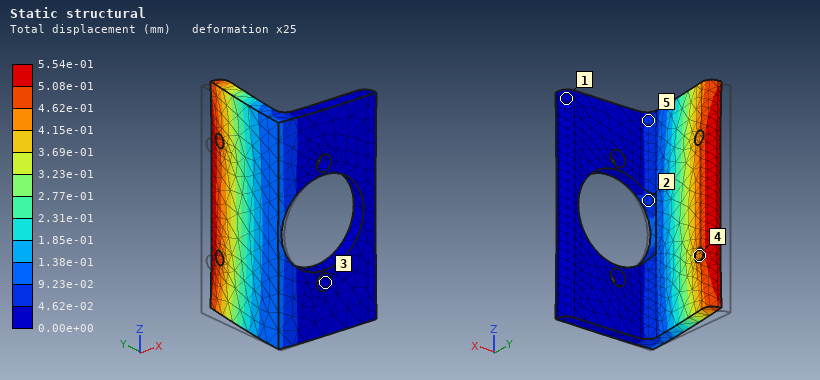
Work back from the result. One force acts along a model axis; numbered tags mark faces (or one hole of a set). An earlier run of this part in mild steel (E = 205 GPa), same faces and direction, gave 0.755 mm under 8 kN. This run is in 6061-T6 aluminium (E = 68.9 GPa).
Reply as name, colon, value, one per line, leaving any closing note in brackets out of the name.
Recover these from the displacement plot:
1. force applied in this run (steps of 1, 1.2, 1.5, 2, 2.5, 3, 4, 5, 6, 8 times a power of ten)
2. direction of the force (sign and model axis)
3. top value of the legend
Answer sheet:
force applied in this run: 2 kN
direction of the force: +X
top value of the legend: 5.54e-01 mm
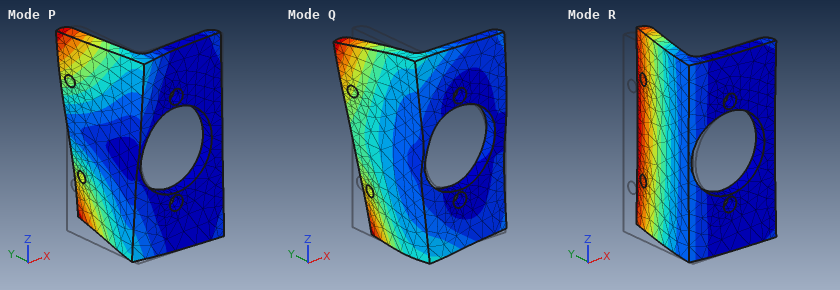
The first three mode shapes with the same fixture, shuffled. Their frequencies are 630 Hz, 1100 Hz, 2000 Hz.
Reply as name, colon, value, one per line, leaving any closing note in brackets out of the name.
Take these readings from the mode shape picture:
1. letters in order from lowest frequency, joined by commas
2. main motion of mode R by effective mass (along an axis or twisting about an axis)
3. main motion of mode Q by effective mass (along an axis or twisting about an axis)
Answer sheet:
letters in order from lowest frequency, joined by commas: R, P, Q
main motion of mode R by effective mass: along X
main motion of mode Q by effective mass: along Z
